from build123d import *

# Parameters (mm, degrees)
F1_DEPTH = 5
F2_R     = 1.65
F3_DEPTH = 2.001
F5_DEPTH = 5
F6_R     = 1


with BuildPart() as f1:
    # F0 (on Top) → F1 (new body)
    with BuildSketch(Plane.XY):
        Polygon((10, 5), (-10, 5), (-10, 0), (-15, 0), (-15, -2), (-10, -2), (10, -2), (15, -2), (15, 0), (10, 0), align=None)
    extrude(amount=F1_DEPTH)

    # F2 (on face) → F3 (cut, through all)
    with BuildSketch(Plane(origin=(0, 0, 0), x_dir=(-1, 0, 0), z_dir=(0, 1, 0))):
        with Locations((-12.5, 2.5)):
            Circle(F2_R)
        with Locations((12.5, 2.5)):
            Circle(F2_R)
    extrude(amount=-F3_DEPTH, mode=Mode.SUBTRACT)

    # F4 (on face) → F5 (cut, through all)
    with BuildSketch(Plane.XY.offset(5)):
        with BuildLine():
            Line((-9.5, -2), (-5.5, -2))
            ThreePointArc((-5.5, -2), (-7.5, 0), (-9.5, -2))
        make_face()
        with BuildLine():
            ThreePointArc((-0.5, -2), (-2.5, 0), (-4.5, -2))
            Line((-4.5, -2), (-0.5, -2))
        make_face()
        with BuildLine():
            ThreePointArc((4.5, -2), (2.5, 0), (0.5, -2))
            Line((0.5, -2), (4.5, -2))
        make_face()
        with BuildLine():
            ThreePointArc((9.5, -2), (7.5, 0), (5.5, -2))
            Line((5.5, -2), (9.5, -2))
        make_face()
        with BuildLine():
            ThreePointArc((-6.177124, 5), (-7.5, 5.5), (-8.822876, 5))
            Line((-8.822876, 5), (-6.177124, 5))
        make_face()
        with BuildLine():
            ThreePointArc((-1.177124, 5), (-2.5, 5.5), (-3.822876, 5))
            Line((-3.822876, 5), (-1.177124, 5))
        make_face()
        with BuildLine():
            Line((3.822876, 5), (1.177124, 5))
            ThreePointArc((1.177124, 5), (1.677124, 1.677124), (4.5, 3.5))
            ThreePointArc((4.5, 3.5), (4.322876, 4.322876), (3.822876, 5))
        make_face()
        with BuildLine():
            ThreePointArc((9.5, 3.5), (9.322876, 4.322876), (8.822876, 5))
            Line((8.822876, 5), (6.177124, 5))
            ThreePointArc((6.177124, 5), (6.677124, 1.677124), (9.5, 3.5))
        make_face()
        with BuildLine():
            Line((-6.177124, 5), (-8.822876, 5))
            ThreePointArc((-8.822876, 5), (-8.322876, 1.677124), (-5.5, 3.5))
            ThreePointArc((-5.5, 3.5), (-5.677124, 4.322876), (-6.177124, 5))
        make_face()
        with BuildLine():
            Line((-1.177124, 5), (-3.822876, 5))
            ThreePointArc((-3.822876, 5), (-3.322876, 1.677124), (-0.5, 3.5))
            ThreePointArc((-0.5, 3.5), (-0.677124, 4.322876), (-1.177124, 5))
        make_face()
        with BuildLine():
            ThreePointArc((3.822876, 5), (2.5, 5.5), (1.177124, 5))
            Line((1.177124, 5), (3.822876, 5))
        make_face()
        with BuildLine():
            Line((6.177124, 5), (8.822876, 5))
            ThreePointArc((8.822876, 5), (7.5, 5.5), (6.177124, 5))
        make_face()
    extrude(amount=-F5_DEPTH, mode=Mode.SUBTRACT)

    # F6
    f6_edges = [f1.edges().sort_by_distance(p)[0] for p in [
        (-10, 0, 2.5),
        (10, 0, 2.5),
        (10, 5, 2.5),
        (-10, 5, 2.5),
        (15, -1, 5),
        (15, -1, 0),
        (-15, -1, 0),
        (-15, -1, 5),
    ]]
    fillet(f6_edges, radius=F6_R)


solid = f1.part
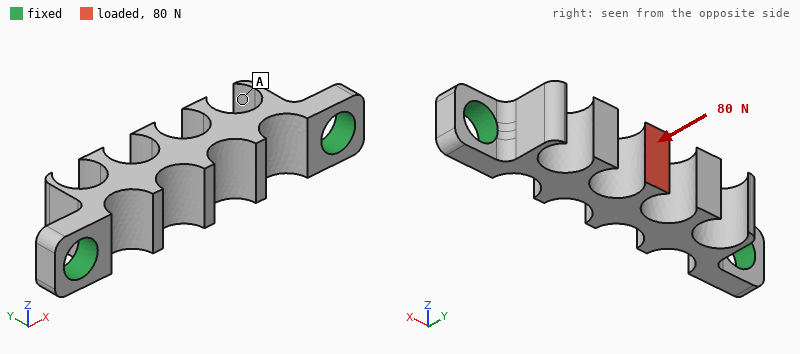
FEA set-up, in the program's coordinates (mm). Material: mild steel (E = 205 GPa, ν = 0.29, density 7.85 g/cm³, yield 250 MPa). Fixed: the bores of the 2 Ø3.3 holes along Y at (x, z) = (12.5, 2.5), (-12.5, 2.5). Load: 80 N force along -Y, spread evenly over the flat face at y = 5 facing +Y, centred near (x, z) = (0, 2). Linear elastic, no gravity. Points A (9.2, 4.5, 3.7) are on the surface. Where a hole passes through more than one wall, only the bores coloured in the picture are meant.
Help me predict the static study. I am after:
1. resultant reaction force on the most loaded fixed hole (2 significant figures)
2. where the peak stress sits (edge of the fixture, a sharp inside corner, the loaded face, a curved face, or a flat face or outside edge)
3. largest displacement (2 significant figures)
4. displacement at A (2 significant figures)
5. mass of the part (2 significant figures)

91 N
a curved face
6.9 µm
2.2 µm
3.2 g
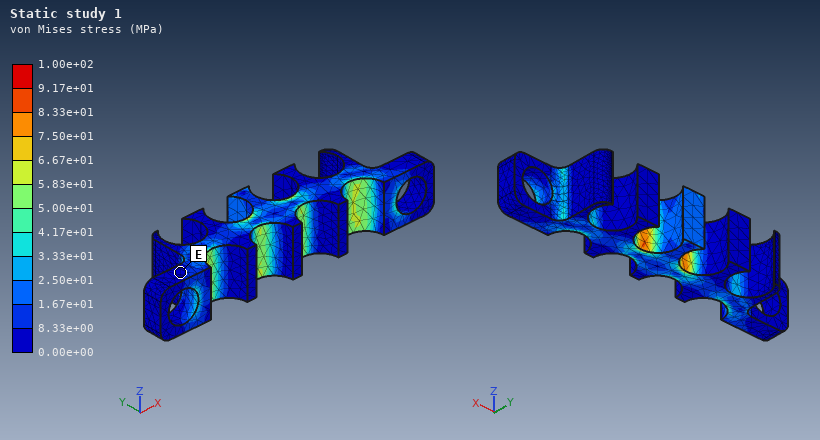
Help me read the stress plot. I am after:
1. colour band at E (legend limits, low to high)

0.00e+00 to 8.33e+00 MPa
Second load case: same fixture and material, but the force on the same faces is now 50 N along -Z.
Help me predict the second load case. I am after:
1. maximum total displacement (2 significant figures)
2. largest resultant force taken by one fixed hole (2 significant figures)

6.9 µm
25 N
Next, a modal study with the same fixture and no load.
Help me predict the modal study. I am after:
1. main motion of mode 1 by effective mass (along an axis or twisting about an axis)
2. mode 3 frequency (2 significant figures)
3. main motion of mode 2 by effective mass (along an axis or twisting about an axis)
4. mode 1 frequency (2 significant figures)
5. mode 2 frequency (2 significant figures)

along Y
30 kHz
along Z
16 kHz
24 kHz
